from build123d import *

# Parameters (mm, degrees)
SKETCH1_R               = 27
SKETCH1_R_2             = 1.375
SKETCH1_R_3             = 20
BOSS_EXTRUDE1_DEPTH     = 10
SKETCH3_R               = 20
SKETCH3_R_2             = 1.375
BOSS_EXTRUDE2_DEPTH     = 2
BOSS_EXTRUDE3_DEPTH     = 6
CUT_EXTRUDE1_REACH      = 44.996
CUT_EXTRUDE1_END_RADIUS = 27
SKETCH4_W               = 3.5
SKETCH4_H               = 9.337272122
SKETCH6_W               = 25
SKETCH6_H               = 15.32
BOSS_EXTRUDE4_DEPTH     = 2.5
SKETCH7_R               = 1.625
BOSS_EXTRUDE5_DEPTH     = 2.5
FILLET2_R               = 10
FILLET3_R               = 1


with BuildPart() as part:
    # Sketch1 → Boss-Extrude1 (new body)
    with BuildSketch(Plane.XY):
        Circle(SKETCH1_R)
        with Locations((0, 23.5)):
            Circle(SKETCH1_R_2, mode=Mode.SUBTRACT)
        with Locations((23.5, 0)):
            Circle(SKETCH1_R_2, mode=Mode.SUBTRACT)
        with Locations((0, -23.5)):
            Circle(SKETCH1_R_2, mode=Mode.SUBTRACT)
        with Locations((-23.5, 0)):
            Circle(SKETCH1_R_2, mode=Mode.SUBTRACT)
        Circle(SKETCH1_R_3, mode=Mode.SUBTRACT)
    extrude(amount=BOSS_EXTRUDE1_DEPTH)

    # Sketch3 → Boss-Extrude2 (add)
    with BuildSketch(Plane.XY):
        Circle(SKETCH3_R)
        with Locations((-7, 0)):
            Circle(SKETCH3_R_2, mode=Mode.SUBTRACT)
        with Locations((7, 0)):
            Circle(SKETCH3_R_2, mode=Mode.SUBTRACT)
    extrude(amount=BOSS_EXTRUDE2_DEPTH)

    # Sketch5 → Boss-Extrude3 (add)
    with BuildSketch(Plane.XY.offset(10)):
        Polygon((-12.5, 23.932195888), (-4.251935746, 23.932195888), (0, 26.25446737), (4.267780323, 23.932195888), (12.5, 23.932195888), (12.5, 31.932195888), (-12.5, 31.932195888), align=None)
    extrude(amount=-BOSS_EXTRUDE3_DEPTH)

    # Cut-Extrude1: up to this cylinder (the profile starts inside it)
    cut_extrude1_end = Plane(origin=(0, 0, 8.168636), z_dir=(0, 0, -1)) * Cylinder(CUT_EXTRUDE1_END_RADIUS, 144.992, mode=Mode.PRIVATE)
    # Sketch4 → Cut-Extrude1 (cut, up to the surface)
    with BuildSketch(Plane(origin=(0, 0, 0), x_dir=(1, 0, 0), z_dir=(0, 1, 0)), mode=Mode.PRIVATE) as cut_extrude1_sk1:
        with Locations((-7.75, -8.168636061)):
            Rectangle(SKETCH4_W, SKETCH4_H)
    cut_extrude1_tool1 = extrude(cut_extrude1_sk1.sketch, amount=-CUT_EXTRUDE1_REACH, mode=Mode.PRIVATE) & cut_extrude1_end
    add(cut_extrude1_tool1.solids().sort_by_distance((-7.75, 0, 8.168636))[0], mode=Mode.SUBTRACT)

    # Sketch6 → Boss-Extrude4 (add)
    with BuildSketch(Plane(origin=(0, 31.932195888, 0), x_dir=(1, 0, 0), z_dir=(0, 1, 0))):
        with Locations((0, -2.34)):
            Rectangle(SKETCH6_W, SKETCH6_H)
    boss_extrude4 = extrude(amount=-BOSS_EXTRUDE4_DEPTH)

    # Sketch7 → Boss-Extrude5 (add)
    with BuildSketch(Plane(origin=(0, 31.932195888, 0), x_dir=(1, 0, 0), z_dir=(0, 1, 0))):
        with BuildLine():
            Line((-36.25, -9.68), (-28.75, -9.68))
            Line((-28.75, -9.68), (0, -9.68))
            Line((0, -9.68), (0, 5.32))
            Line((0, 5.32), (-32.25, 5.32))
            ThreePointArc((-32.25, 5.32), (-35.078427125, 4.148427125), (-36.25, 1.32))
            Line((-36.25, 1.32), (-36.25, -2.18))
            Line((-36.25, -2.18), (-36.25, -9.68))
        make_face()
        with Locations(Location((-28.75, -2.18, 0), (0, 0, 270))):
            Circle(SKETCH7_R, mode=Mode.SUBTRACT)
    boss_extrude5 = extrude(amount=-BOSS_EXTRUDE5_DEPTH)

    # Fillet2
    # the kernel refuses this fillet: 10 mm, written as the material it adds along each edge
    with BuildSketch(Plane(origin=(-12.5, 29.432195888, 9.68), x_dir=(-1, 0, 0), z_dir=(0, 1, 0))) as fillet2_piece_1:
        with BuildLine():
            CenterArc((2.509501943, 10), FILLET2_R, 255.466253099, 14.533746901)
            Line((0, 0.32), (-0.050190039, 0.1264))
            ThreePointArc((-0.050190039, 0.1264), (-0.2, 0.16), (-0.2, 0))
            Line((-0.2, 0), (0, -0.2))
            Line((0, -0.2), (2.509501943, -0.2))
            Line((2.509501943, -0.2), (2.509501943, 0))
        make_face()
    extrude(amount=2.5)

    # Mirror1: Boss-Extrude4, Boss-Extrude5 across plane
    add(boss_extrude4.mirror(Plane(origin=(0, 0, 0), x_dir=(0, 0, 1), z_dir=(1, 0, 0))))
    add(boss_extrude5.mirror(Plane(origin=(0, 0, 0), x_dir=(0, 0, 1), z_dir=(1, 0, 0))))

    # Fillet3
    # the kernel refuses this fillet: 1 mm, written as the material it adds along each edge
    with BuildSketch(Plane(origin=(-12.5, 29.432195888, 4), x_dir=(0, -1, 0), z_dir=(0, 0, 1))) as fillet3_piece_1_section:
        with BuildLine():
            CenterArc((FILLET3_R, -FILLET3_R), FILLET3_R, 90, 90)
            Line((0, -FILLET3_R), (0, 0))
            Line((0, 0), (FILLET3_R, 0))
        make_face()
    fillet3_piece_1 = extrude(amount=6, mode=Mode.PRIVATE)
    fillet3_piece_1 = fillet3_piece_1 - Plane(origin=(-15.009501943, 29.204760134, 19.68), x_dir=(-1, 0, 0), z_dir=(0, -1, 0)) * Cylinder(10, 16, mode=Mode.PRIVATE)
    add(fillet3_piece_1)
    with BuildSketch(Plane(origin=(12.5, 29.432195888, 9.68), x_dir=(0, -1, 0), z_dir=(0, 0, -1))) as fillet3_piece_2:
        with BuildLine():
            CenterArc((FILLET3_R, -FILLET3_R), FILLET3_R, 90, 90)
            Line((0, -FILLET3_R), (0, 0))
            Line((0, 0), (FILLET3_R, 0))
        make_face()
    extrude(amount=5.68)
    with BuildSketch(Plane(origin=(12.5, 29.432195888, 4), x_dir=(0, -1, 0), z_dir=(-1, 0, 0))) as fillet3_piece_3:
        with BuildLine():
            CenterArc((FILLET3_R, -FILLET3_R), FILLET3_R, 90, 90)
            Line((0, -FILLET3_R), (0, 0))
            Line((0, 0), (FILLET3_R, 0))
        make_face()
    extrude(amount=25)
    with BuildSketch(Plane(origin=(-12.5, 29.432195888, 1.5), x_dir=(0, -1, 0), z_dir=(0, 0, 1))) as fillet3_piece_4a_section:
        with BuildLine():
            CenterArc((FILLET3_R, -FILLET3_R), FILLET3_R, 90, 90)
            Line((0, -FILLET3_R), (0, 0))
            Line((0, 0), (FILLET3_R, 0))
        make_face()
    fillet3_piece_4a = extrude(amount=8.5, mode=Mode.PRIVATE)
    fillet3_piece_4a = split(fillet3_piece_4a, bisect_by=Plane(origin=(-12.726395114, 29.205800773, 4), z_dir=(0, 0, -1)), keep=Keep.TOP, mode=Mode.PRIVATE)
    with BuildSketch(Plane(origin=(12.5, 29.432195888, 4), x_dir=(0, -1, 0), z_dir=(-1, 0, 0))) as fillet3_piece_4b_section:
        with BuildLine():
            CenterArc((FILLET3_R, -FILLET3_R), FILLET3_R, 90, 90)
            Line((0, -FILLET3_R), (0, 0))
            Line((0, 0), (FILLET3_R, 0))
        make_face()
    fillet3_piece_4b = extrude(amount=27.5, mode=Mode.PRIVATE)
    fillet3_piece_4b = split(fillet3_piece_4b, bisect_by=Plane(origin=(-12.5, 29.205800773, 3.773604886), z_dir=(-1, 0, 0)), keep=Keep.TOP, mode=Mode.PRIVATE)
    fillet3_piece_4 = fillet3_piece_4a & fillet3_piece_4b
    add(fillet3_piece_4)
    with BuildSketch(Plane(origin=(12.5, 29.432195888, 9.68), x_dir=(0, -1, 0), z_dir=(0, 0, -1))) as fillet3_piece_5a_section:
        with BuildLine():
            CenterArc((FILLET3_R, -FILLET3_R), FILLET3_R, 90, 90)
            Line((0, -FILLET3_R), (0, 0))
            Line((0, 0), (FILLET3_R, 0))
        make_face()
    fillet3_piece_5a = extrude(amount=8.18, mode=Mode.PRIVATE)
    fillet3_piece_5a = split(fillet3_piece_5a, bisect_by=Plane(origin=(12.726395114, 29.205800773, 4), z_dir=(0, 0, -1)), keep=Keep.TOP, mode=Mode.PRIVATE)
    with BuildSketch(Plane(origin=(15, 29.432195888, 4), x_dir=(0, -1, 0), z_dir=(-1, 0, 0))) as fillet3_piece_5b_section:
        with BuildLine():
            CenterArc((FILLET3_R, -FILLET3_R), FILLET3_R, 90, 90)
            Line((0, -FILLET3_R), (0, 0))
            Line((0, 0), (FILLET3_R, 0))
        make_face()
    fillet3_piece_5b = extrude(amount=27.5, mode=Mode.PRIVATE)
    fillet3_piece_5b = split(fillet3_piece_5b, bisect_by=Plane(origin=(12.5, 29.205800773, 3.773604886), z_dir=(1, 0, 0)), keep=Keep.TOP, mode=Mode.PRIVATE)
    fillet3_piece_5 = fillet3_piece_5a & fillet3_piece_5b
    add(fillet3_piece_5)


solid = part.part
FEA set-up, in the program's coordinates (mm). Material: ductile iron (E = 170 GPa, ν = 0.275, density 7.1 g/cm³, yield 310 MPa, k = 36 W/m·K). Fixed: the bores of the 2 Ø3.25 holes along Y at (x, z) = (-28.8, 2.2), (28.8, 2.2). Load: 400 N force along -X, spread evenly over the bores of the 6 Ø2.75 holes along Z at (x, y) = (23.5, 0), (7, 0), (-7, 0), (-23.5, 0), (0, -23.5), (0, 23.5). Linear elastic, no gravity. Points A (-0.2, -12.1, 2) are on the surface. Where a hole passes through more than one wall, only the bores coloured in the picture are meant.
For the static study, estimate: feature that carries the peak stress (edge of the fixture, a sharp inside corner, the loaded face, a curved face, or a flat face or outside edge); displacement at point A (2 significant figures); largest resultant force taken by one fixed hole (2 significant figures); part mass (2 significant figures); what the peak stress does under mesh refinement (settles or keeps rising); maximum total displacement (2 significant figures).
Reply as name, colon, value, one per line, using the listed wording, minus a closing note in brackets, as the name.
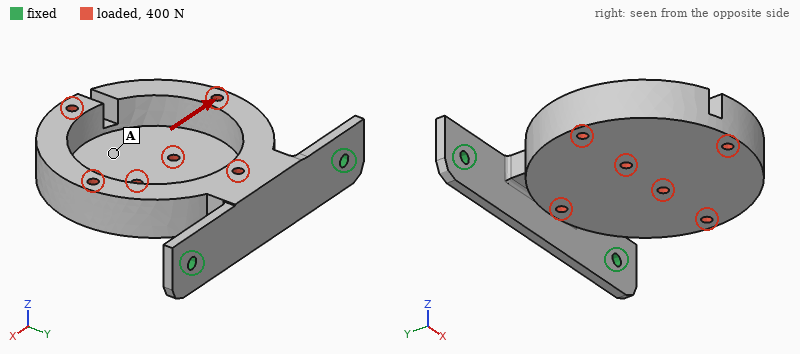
feature that carries the peak stress: a sharp inside corner
displacement at point A: 0.12 mm
largest resultant force taken by one fixed hole: 350 N
part mass: 110 g
what the peak stress does under mesh refinement: keeps rising
maximum total displacement: 0.16 mm
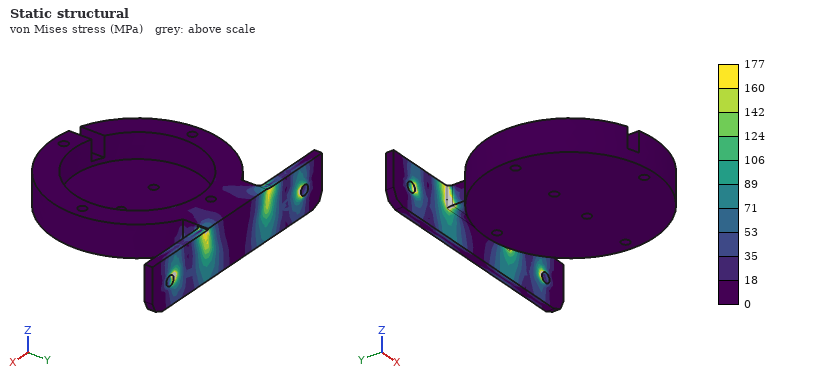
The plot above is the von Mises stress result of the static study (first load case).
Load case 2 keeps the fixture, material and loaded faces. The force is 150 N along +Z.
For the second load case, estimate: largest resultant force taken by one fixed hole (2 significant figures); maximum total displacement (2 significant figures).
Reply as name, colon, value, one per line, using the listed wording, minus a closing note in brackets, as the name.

largest resultant force taken by one fixed hole: 75 N
maximum total displacement: 0.53 mm
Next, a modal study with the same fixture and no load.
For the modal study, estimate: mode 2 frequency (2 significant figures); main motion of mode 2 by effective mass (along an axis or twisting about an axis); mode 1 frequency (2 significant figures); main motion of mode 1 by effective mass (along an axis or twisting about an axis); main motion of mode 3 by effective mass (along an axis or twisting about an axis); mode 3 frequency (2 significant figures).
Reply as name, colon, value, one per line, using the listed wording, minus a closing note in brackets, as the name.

mode 2 frequency: 950 Hz
main motion of mode 2 by effective mass: along X
mode 1 frequency: 350 Hz
main motion of mode 1 by effective mass: along Z
main motion of mode 3 by effective mass: along Y
mode 3 frequency: 1700 Hz
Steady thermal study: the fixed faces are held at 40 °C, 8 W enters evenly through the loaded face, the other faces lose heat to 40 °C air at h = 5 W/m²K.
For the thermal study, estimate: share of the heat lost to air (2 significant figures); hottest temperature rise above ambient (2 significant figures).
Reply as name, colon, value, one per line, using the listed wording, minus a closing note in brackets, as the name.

share of the heat lost to air: 32 %
hottest temperature rise above ambient: 75 K
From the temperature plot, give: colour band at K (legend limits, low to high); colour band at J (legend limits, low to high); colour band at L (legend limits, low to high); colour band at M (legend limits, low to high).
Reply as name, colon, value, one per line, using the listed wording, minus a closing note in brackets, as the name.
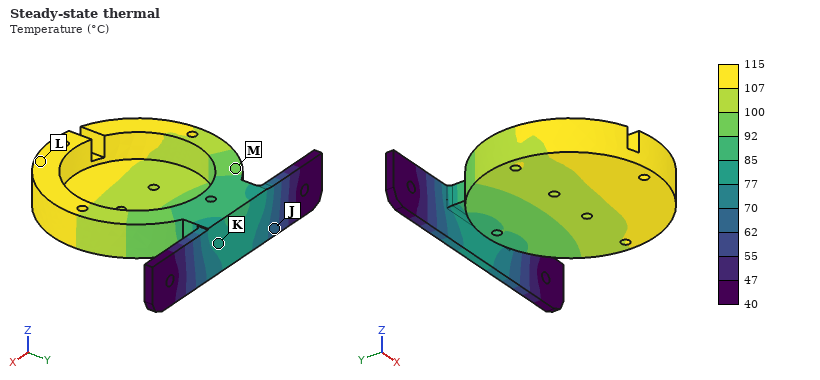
colour band at K: 77 to 85 °C
colour band at J: 62 to 70 °C
colour band at L: 107 to 115 °C
colour band at M: 92 to 100 °C
